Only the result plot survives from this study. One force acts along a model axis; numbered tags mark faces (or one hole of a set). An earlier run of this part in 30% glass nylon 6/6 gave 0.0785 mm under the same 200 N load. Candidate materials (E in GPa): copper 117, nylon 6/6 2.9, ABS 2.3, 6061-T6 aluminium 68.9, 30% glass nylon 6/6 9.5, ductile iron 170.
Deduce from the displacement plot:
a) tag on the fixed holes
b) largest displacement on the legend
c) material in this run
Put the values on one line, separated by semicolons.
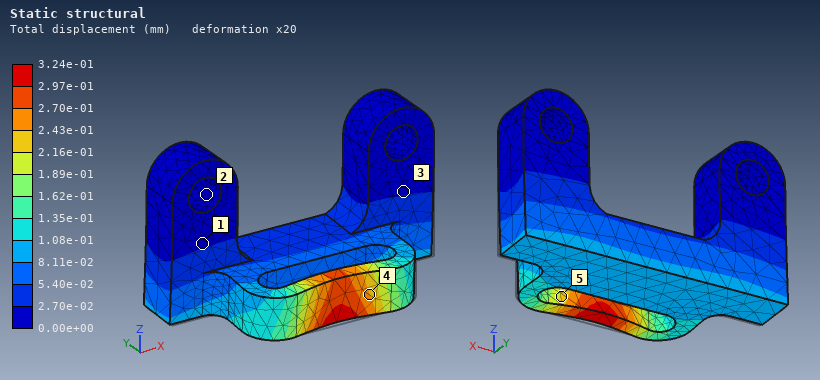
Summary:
2; 3.24e-01 mm; ABS
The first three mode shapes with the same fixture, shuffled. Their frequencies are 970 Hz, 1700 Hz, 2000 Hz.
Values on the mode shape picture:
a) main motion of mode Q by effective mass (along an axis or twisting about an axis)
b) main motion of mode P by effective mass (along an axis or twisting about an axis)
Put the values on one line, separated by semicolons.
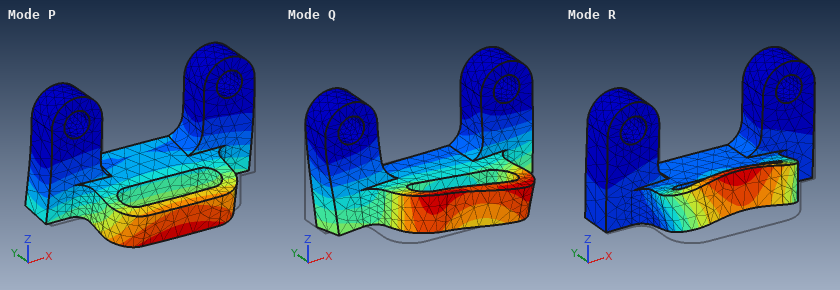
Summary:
along X; along Y
